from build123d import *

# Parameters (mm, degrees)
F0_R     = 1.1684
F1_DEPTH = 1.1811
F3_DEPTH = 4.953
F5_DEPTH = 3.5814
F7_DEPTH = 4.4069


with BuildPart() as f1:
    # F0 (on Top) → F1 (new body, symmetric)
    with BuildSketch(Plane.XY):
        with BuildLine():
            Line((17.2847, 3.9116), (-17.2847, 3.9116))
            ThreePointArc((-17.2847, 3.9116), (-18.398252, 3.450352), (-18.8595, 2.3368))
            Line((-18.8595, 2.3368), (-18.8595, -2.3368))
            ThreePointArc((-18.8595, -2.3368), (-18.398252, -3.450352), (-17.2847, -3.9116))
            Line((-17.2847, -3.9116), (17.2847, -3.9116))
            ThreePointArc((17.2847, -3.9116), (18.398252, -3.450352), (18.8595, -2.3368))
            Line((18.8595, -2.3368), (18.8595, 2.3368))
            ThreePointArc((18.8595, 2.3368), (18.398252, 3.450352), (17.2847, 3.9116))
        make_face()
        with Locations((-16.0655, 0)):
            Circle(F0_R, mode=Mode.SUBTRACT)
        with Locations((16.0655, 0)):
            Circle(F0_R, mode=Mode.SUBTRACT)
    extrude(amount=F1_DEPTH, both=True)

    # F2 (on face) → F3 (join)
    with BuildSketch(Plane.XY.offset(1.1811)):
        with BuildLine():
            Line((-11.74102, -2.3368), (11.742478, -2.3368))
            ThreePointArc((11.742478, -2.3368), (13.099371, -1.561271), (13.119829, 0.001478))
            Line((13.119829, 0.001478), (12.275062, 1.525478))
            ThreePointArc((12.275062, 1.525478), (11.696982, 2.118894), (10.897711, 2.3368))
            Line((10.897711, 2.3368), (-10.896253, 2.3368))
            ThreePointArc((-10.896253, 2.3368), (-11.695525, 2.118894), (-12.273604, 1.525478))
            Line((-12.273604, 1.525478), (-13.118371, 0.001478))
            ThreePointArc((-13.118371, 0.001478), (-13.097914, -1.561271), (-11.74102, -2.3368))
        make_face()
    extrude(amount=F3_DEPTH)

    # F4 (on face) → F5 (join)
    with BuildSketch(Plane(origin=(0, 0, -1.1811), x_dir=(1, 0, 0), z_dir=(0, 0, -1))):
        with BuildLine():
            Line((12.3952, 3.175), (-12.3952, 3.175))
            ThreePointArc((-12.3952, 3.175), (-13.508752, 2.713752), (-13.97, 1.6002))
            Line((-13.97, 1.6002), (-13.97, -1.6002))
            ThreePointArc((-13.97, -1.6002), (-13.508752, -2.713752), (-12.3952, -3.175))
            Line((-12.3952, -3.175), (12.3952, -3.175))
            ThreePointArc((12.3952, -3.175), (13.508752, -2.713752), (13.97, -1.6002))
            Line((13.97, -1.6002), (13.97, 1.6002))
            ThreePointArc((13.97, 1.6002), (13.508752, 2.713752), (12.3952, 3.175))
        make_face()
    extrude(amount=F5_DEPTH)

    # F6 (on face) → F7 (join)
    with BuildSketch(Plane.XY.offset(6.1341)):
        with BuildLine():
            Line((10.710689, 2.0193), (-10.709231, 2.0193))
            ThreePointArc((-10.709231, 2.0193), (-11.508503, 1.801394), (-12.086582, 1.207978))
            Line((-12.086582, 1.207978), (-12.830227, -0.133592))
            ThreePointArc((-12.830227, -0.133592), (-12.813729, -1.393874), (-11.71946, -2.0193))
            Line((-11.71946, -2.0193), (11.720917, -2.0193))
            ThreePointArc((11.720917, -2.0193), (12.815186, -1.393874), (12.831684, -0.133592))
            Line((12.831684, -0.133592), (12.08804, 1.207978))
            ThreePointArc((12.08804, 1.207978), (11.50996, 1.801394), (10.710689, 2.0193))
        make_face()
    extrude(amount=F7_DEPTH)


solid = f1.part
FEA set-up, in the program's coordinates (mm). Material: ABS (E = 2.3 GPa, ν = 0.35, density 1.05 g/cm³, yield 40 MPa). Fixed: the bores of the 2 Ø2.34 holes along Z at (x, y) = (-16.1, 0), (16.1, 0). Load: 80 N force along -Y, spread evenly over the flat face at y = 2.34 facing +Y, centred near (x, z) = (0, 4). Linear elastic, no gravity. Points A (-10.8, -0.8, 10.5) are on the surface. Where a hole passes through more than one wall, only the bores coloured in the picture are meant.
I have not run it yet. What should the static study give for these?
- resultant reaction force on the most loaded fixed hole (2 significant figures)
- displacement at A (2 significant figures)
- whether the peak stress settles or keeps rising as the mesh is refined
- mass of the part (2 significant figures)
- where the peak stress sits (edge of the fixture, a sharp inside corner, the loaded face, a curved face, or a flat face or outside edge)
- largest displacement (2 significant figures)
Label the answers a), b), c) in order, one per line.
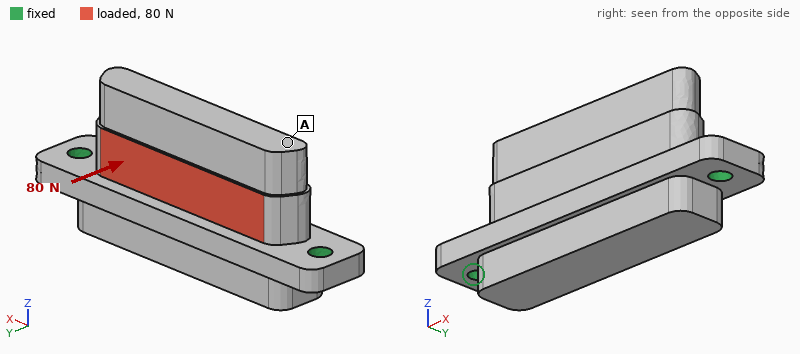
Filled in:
a) 40 N
b) 0.21 mm
c) keeps rising
d) 2.4 g
e) edge of the fixture
f) 0.25 mm
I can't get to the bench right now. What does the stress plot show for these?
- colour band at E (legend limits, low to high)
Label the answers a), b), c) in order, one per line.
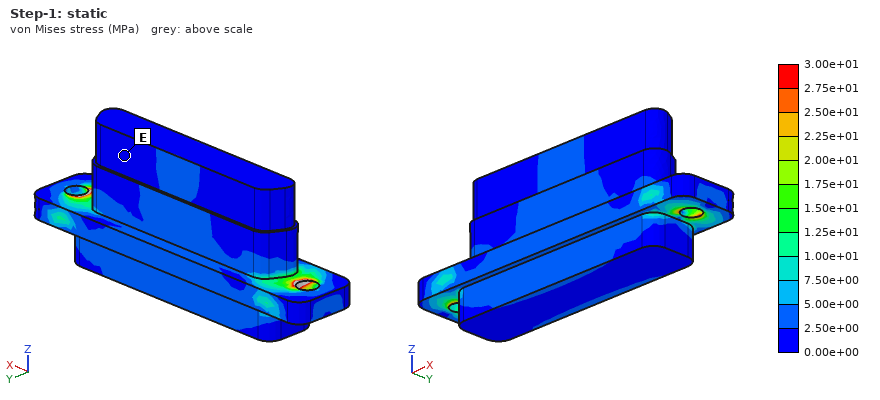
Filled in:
a) 0.00e+00 to 2.50e+00 MPa
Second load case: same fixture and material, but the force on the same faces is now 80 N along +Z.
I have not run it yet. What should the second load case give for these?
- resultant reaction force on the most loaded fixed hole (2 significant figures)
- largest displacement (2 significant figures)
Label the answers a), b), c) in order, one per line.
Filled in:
a) 40 N
b) 0.13 mm
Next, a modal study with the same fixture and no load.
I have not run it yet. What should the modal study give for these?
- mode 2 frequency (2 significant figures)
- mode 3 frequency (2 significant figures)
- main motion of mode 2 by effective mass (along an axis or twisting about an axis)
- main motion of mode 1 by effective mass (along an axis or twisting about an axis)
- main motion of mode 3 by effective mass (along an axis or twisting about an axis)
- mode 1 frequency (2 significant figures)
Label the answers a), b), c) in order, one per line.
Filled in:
a) 5100 Hz
b) 6000 Hz
c) along Y
d) along Y
e) along Z
f) 2700 Hz
